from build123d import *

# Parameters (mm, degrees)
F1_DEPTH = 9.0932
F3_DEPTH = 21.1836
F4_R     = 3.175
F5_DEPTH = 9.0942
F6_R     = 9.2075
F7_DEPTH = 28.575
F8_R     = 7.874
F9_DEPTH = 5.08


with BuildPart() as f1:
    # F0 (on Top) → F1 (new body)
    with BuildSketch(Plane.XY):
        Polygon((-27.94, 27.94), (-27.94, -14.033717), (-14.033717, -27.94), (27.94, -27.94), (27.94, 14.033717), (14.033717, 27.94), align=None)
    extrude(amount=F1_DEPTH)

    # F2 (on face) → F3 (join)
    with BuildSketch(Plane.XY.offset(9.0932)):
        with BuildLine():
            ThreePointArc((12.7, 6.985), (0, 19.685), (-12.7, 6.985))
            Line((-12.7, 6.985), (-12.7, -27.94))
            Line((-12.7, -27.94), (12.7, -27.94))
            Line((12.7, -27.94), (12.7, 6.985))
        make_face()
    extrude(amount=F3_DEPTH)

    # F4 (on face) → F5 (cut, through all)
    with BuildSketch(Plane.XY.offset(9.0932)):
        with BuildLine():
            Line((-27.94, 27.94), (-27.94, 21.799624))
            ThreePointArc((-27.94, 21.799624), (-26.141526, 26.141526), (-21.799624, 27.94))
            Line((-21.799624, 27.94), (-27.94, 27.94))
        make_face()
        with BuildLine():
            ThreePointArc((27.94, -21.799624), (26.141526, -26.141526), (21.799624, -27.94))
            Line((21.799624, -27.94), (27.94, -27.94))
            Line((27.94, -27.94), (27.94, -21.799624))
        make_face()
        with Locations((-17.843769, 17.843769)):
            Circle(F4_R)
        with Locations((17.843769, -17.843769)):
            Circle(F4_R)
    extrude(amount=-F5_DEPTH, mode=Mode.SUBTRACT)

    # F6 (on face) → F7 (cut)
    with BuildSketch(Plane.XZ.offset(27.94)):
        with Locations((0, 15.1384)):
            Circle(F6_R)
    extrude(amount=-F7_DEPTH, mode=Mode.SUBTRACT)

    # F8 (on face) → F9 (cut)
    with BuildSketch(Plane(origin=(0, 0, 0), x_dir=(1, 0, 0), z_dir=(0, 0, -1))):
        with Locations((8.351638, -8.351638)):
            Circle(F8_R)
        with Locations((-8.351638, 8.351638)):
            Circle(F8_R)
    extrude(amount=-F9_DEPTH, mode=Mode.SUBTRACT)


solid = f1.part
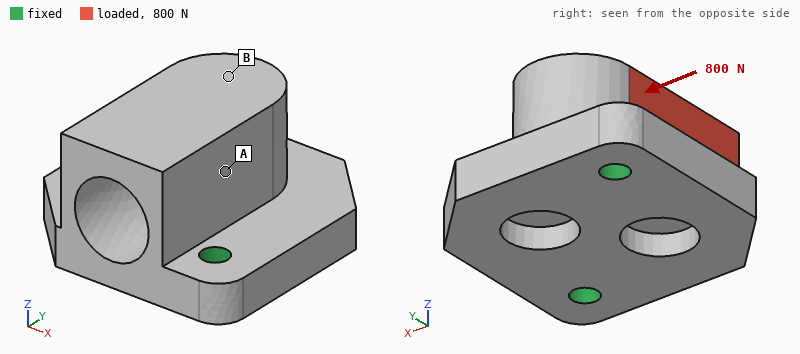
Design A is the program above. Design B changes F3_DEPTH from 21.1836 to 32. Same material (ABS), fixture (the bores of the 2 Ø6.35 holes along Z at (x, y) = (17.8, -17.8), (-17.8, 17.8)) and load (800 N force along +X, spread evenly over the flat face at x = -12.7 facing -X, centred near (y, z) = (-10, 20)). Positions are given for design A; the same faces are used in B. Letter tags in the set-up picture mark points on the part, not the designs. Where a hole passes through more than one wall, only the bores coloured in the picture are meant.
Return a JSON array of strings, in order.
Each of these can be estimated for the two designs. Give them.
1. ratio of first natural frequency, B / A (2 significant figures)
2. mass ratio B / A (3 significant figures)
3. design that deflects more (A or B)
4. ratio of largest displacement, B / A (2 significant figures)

["0.67", "1.30", "B", "1.6"]
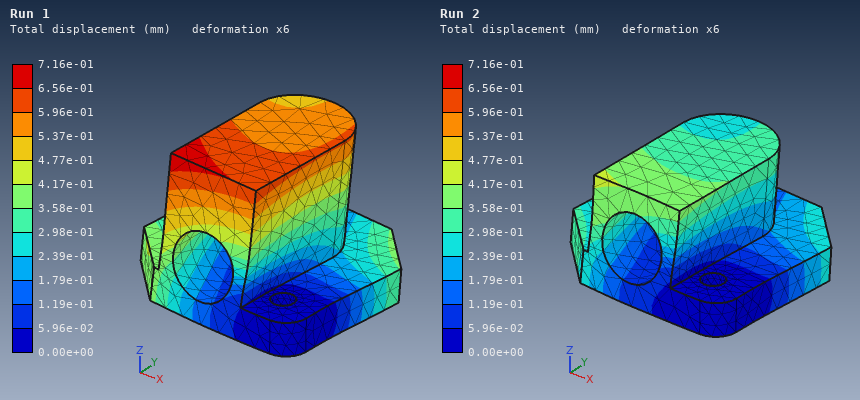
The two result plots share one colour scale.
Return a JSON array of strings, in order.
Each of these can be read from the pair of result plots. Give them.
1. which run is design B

["Run 1"]
